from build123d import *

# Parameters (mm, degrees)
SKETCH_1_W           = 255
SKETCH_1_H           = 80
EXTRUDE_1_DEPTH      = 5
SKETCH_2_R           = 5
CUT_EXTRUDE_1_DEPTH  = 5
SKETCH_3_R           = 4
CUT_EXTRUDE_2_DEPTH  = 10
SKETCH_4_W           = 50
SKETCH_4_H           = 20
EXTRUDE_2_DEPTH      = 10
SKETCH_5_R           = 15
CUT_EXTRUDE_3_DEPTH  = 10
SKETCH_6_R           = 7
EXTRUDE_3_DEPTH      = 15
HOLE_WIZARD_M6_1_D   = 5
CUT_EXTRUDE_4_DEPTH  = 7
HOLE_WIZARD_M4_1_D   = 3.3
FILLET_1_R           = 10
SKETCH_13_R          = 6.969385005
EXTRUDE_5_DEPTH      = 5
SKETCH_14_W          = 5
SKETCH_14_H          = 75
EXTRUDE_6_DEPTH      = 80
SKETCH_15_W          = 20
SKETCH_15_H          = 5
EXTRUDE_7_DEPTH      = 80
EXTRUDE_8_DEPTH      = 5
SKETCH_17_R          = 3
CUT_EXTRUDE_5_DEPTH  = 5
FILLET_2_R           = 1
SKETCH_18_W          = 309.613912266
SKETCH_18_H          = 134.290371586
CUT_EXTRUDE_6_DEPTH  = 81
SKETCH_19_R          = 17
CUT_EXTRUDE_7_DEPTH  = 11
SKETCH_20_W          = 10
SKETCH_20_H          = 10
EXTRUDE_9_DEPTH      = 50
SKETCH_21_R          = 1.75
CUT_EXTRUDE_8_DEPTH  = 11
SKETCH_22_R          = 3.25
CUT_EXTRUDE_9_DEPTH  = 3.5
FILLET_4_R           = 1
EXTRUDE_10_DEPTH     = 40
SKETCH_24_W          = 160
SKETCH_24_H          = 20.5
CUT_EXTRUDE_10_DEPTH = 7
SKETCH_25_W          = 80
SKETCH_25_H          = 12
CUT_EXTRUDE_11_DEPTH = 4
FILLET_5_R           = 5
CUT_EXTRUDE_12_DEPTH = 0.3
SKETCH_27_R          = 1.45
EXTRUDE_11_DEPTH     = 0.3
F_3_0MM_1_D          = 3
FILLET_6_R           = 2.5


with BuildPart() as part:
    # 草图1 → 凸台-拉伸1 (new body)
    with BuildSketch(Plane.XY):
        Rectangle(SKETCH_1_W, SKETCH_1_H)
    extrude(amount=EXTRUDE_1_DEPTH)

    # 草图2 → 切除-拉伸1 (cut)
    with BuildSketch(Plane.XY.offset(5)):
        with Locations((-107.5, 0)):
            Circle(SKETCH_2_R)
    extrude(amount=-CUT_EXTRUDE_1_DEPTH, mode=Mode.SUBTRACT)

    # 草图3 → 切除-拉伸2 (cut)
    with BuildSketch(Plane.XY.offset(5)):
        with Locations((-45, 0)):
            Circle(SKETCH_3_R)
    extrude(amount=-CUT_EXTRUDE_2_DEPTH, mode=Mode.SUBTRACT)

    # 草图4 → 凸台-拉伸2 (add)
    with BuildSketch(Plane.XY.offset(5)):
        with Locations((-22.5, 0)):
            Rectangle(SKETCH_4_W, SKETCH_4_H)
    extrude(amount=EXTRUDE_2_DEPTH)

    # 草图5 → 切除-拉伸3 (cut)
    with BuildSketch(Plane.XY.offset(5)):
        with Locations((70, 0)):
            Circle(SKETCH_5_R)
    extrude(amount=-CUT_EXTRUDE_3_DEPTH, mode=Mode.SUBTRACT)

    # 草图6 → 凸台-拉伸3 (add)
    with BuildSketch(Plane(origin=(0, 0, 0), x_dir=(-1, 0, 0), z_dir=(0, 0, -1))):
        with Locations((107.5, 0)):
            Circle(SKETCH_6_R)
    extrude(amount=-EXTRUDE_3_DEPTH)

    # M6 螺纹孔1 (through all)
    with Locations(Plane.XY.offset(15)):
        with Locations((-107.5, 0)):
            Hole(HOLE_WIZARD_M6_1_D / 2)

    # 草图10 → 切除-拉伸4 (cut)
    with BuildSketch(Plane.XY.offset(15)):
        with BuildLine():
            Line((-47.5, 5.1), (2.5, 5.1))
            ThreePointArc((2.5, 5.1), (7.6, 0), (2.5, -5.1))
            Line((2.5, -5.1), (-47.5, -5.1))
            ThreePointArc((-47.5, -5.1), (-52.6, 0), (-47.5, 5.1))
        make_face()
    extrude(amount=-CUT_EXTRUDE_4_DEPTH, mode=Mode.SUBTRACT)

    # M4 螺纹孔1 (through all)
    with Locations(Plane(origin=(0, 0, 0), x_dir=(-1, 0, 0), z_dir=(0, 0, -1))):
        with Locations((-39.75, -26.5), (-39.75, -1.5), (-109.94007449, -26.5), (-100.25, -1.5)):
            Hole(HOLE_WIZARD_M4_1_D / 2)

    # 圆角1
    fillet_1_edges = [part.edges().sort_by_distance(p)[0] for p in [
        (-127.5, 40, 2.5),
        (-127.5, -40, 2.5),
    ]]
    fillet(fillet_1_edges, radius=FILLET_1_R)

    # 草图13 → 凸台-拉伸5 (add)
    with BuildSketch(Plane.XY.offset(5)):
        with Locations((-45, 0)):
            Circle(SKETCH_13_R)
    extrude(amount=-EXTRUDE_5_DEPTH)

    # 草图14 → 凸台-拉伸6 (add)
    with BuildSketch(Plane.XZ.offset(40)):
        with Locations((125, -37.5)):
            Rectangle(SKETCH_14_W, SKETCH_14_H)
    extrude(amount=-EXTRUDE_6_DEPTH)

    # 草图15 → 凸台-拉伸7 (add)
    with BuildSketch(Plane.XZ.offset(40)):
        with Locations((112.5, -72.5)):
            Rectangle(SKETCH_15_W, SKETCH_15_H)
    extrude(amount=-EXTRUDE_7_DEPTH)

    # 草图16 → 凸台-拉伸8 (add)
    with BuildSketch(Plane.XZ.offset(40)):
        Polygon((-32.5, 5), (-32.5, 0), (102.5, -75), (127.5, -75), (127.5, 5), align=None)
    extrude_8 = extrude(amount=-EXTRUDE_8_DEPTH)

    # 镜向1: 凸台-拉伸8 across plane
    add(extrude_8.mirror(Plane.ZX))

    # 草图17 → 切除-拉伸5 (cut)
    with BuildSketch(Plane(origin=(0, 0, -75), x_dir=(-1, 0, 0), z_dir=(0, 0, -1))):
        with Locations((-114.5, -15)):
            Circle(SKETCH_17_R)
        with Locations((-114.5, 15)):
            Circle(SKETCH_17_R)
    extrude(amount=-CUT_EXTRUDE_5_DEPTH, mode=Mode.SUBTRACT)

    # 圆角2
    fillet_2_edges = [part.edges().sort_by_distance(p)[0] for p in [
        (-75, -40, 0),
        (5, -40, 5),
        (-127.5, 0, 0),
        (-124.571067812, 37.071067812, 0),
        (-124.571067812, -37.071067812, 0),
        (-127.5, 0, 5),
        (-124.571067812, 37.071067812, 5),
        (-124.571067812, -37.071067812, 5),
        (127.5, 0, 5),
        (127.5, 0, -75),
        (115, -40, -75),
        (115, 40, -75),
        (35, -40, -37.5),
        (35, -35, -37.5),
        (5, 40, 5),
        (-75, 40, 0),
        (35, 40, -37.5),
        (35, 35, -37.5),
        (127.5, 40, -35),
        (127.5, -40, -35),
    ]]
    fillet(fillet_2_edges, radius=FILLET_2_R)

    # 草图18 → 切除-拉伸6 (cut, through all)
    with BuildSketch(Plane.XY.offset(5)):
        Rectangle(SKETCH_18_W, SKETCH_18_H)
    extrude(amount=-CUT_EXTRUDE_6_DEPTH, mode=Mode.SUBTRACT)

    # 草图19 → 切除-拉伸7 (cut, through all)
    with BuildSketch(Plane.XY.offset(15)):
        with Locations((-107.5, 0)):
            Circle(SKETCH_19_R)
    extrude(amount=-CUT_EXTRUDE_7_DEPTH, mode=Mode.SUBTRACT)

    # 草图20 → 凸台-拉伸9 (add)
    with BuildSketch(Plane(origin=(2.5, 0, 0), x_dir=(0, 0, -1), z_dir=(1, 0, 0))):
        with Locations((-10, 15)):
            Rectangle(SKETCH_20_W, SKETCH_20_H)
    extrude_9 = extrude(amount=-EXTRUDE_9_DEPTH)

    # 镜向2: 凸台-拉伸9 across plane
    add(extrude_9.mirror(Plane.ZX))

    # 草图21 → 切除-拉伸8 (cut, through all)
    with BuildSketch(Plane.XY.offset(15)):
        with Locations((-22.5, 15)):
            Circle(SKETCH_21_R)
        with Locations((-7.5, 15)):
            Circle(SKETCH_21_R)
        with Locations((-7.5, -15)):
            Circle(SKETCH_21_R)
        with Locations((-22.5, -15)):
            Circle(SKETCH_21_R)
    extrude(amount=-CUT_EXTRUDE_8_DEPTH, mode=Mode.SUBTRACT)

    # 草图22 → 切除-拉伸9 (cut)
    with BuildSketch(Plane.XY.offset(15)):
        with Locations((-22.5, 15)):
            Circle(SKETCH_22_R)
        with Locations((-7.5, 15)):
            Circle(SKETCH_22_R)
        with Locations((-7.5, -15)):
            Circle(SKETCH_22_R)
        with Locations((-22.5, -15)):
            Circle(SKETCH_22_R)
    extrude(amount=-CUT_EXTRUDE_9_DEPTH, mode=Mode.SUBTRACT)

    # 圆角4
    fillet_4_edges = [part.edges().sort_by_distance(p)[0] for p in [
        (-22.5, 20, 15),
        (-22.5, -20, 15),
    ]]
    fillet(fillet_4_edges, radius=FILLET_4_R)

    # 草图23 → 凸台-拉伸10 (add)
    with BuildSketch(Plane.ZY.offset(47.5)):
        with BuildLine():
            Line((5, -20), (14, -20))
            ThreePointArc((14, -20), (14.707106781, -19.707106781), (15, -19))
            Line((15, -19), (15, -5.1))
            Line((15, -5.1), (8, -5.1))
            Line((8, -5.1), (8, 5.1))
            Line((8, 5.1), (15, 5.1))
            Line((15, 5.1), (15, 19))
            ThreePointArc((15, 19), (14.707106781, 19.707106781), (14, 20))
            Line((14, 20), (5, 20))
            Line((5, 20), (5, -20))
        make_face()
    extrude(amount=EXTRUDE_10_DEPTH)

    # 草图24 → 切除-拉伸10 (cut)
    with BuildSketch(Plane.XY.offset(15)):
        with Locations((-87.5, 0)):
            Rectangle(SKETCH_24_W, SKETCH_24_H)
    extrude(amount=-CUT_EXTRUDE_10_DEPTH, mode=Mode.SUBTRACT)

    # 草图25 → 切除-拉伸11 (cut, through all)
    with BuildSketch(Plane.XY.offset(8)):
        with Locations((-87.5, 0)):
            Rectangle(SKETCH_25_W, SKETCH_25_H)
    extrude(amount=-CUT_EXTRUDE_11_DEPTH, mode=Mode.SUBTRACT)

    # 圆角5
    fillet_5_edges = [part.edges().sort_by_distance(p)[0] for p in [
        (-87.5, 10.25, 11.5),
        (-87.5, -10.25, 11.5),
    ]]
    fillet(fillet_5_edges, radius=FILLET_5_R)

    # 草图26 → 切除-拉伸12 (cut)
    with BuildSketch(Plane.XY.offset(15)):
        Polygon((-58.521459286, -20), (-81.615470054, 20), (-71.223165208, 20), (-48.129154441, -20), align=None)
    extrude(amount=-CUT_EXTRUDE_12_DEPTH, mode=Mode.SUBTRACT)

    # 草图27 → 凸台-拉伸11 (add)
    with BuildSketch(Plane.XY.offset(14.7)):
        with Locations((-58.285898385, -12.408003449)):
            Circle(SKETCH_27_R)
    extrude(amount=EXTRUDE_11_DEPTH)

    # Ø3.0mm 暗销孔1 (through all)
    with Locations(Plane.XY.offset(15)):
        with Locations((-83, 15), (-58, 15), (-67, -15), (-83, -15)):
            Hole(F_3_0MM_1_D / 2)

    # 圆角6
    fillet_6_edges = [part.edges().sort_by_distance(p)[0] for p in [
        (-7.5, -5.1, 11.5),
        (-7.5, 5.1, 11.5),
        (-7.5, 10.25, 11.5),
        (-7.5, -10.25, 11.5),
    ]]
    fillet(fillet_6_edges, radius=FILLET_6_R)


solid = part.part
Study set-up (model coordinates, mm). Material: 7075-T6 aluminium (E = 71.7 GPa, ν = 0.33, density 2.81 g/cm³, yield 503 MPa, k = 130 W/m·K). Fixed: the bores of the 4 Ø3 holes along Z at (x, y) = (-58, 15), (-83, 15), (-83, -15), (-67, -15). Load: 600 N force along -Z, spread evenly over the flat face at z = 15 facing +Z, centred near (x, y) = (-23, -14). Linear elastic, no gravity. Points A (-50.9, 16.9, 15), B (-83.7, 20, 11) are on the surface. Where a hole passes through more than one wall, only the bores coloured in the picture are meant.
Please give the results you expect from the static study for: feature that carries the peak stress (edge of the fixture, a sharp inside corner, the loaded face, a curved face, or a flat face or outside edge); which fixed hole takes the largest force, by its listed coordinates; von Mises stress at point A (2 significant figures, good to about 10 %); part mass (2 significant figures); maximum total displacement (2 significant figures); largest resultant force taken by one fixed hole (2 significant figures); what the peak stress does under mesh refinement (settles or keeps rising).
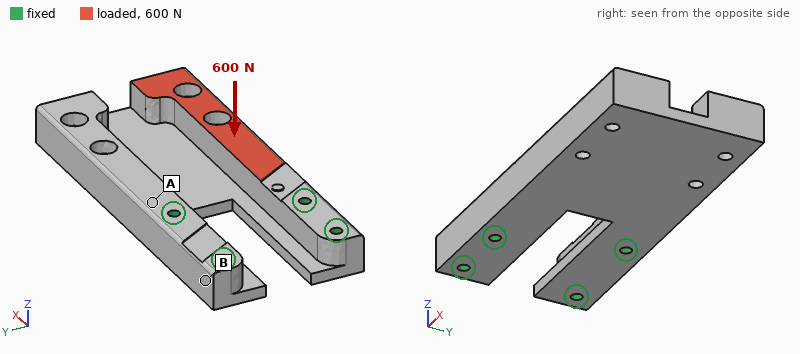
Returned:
edge of the fixture
(-67, -15)
51 MPa
60 g
0.30 mm
590 N
keeps rising
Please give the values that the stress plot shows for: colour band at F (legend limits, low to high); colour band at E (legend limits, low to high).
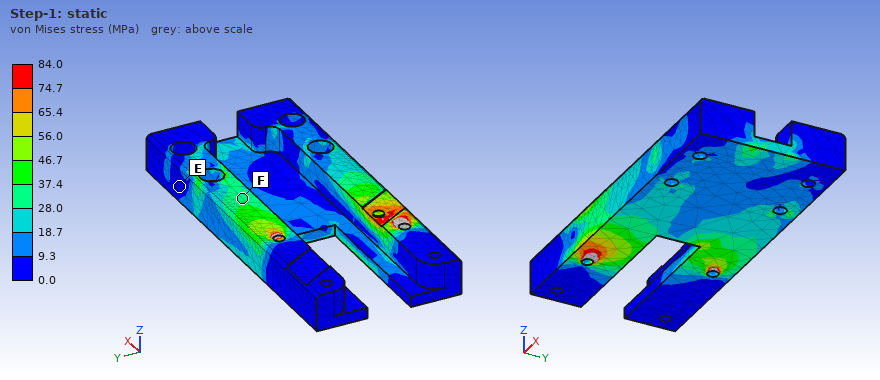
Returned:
28.0 to 37.4 MPa
0.0 to 9.3 MPa
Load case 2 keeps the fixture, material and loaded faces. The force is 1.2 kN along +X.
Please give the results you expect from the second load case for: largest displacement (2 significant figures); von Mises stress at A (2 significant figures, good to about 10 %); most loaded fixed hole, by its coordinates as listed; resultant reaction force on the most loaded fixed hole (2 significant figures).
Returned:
0.12 mm
17 MPa
(-67, -15)
1.1 kN
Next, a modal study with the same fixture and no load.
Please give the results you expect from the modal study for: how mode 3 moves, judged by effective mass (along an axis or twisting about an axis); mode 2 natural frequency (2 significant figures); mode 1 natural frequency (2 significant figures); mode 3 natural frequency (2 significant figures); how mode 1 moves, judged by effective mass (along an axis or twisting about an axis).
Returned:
along Y
3400 Hz
1700 Hz
5600 Hz
along Z
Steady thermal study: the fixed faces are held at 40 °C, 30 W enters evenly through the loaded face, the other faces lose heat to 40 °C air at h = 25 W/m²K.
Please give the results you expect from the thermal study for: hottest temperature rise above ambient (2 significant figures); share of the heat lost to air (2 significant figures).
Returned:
44 K
15 %
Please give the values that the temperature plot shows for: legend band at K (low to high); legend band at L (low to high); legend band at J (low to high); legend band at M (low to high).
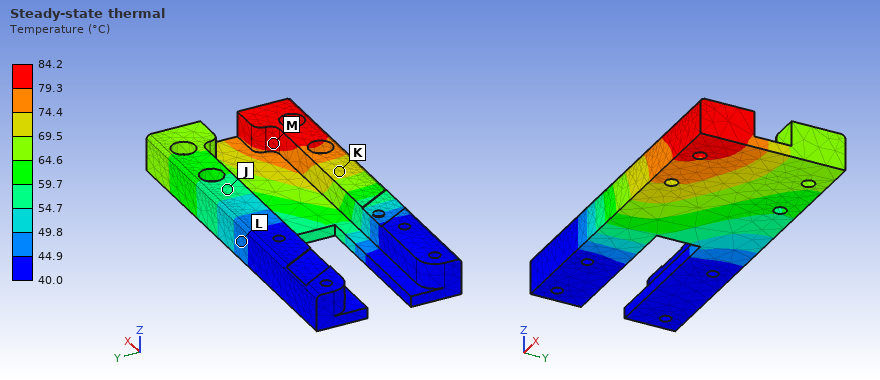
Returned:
69.5 to 74.4 °C
44.9 to 49.8 °C
54.7 to 59.7 °C
79.3 to 84.2 °C
